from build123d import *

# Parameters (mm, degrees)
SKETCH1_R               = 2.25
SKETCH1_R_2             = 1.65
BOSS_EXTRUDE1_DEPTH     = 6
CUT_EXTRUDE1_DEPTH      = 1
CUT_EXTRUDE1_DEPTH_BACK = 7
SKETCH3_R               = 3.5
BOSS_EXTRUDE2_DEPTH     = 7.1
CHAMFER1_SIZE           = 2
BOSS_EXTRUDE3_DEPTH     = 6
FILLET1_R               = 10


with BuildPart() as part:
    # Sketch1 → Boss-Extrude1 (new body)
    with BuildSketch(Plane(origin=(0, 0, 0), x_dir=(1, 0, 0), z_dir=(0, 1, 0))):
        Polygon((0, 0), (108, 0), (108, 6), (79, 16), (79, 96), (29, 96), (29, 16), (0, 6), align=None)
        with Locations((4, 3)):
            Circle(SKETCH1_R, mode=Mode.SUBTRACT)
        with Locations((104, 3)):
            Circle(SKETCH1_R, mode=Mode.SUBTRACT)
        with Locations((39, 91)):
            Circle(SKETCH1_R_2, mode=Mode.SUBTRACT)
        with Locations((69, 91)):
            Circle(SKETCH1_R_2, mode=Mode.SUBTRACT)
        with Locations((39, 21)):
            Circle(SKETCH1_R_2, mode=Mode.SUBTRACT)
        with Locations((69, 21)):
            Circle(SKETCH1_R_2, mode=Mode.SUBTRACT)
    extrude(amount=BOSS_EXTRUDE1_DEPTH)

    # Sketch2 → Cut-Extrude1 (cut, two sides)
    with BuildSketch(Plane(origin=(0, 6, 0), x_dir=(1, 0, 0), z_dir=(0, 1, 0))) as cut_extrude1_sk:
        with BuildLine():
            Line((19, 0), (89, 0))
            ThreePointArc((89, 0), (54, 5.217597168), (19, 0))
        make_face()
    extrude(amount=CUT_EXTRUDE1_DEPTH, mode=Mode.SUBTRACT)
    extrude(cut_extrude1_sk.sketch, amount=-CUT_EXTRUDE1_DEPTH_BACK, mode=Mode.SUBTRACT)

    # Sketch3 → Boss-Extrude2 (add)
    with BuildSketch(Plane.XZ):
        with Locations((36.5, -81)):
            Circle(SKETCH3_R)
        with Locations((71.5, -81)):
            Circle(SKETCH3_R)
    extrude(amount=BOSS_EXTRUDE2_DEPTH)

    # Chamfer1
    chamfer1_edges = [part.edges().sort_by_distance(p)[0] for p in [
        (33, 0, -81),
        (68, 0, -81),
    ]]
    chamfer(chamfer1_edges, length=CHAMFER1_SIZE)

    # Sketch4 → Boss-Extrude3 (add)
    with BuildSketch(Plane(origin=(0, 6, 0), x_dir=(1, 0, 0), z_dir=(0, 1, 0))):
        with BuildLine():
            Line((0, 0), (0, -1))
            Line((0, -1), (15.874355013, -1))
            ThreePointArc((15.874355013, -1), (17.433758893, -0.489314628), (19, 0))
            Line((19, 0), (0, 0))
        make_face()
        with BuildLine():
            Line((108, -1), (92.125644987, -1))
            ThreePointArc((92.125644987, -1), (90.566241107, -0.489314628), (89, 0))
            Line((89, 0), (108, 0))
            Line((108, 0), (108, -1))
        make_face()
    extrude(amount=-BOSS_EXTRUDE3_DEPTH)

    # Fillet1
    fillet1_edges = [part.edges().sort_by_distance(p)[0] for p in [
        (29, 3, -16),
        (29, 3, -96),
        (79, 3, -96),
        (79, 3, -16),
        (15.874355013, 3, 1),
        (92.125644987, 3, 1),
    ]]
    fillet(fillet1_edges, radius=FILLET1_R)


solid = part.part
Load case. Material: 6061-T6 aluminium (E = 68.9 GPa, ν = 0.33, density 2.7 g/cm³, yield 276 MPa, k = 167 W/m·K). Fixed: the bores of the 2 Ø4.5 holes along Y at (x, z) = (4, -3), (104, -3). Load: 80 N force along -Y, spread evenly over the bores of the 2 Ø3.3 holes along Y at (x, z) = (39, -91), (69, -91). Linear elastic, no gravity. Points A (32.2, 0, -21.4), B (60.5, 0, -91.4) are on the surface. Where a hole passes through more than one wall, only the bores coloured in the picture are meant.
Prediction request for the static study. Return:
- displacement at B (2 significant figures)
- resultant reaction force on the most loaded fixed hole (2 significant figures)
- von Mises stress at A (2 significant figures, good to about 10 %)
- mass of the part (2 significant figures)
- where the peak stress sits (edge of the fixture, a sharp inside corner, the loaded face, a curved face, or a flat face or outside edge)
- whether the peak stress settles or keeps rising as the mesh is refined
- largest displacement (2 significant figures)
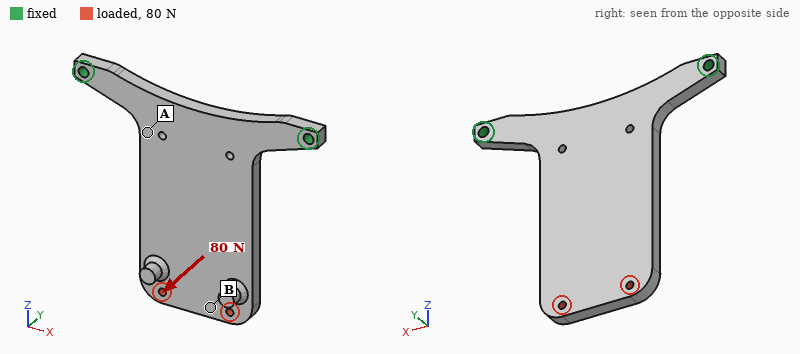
0.81 mm
40 N
26 MPa
85 g
edge of the fixture
keeps rising
0.86 mm
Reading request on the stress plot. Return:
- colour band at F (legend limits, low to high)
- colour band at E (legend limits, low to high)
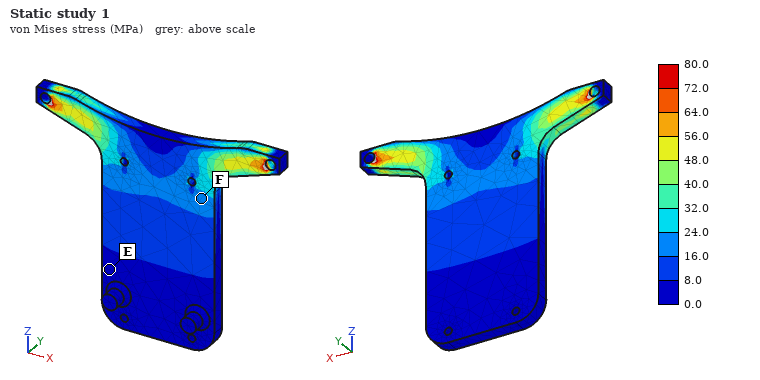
16.0 to 24.0 MPa
0.0 to 8.0 MPa
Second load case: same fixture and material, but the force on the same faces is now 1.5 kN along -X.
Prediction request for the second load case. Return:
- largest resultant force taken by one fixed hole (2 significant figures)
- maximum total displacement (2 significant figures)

1.7 kN
0.27 mm
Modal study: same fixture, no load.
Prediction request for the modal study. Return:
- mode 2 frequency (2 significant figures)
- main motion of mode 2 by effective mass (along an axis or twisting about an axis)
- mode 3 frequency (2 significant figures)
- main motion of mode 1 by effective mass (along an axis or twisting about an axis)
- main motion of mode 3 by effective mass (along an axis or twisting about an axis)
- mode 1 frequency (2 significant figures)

2000 Hz
twisting about Z
2100 Hz
along Y
along Y
310 Hz
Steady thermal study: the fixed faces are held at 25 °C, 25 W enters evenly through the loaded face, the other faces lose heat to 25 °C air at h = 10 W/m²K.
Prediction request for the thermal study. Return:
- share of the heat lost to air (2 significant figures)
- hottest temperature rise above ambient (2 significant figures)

20 %
65 K
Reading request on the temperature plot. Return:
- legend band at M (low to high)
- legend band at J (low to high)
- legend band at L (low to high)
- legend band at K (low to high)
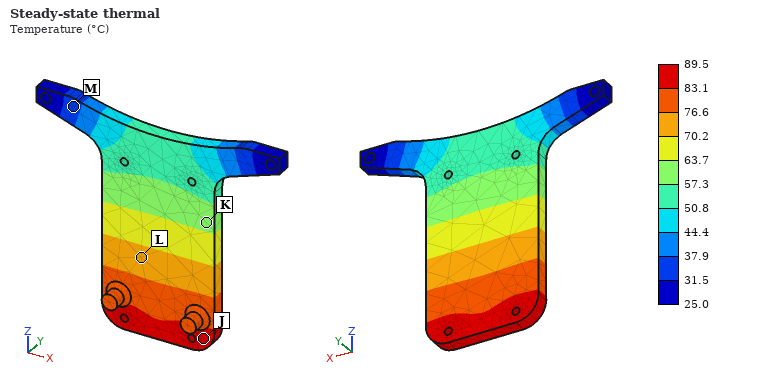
31.5 to 37.9 °C
83.1 to 89.5 °C
70.2 to 76.6 °C
57.3 to 63.7 °C
